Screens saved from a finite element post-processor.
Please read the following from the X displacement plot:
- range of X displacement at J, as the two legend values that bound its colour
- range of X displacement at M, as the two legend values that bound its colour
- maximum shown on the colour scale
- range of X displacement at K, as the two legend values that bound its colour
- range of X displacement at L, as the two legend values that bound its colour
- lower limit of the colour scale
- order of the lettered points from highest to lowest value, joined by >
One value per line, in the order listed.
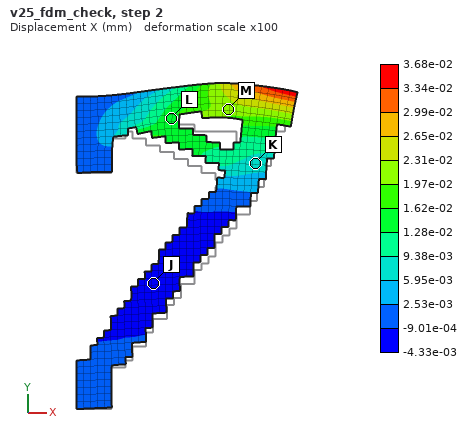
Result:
-4.33e-03 to -9.01e-04 mm
1.97e-02 to 2.31e-02 mm
3.68e-02 mm
5.95e-03 to 9.38e-03 mm
1.28e-02 to 1.62e-02 mm
-4.33e-03 mm
M > L > K > J
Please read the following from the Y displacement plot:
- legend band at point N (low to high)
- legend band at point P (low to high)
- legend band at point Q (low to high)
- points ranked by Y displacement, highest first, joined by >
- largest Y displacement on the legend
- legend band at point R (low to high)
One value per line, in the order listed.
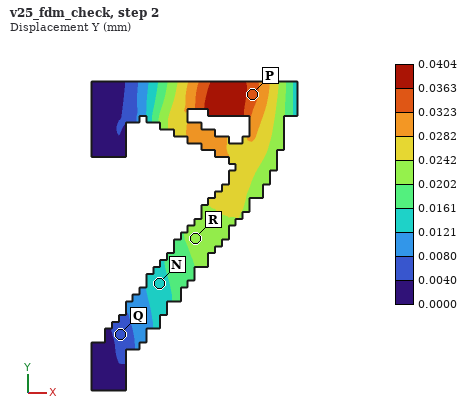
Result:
0.0121 to 0.0161 mm
0.0323 to 0.0363 mm
0.0040 to 0.0080 mm
P > R > N > Q
0.0404 mm
0.0202 to 0.0242 mm
